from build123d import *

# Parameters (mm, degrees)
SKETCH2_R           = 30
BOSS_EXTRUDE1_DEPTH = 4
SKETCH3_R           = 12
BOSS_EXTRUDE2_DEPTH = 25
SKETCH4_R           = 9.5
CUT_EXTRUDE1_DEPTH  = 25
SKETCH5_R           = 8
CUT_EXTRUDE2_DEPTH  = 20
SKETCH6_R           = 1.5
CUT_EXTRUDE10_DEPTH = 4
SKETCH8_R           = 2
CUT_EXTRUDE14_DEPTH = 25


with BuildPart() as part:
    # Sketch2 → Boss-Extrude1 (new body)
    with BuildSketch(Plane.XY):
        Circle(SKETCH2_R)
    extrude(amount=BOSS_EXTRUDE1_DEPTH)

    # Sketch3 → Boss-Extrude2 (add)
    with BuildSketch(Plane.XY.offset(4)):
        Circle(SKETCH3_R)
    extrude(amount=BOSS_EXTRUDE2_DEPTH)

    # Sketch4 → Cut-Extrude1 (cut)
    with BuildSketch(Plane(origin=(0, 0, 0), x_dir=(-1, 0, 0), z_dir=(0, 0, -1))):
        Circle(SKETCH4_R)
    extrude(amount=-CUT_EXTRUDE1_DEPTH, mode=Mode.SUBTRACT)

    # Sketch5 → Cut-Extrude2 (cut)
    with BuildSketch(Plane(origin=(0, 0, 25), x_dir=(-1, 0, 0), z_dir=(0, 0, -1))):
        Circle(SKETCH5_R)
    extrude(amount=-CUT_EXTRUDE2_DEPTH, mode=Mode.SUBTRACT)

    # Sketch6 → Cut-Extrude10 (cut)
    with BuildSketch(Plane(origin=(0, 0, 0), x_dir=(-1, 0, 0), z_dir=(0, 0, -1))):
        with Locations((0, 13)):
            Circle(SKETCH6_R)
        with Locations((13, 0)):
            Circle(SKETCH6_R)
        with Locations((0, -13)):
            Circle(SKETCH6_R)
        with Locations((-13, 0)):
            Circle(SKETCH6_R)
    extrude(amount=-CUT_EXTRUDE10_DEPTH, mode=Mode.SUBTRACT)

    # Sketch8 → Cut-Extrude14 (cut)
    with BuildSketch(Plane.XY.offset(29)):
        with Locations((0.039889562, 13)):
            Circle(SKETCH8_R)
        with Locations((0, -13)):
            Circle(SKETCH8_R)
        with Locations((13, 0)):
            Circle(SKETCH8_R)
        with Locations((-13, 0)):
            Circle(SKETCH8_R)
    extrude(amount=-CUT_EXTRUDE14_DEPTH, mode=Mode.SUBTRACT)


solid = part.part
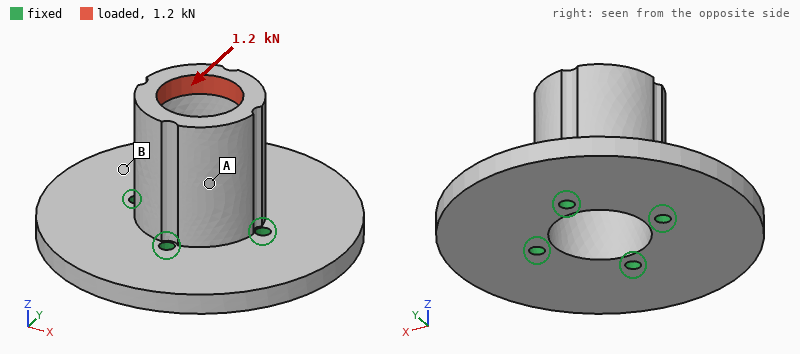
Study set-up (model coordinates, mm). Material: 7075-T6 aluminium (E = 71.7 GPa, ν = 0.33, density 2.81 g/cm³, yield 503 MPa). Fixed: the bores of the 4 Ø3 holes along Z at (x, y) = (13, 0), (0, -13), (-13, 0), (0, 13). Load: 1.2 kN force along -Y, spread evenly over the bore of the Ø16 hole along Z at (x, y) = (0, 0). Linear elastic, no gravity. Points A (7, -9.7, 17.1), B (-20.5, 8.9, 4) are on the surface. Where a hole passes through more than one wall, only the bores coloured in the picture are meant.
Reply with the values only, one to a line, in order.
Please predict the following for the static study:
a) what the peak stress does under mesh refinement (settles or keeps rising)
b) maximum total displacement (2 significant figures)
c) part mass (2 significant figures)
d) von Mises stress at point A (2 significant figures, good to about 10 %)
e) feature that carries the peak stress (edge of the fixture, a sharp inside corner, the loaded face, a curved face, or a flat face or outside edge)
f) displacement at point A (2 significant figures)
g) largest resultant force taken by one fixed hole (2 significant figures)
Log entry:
keeps rising
35 µm
40 g
18 MPa
edge of the fixture
17 µm
1.2 kN
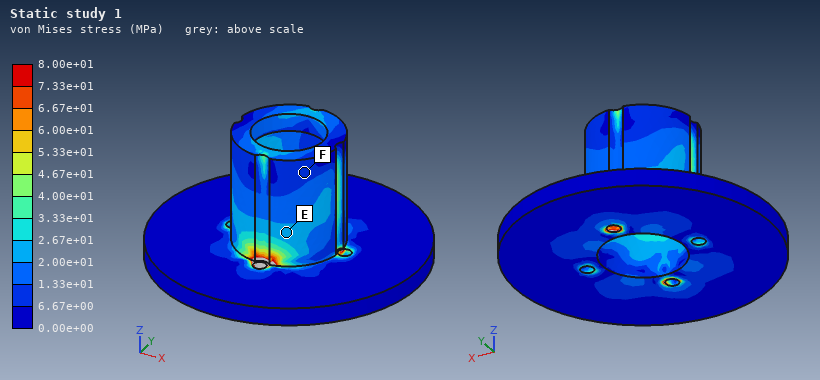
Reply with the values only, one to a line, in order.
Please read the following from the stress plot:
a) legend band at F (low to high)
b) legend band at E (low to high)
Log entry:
6.67e+00 to 1.33e+01 MPa
2.00e+01 to 2.67e+01 MPa
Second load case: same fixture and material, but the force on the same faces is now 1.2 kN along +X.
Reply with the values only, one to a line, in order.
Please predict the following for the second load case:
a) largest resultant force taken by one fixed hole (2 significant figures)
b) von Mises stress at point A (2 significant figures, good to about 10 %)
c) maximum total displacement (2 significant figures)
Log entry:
1.2 kN
20 MPa
35 µm
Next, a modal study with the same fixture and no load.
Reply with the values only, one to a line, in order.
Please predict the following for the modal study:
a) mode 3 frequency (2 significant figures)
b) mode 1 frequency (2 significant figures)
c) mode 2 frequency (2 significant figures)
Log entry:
8700 Hz
8400 Hz
8700 Hz
